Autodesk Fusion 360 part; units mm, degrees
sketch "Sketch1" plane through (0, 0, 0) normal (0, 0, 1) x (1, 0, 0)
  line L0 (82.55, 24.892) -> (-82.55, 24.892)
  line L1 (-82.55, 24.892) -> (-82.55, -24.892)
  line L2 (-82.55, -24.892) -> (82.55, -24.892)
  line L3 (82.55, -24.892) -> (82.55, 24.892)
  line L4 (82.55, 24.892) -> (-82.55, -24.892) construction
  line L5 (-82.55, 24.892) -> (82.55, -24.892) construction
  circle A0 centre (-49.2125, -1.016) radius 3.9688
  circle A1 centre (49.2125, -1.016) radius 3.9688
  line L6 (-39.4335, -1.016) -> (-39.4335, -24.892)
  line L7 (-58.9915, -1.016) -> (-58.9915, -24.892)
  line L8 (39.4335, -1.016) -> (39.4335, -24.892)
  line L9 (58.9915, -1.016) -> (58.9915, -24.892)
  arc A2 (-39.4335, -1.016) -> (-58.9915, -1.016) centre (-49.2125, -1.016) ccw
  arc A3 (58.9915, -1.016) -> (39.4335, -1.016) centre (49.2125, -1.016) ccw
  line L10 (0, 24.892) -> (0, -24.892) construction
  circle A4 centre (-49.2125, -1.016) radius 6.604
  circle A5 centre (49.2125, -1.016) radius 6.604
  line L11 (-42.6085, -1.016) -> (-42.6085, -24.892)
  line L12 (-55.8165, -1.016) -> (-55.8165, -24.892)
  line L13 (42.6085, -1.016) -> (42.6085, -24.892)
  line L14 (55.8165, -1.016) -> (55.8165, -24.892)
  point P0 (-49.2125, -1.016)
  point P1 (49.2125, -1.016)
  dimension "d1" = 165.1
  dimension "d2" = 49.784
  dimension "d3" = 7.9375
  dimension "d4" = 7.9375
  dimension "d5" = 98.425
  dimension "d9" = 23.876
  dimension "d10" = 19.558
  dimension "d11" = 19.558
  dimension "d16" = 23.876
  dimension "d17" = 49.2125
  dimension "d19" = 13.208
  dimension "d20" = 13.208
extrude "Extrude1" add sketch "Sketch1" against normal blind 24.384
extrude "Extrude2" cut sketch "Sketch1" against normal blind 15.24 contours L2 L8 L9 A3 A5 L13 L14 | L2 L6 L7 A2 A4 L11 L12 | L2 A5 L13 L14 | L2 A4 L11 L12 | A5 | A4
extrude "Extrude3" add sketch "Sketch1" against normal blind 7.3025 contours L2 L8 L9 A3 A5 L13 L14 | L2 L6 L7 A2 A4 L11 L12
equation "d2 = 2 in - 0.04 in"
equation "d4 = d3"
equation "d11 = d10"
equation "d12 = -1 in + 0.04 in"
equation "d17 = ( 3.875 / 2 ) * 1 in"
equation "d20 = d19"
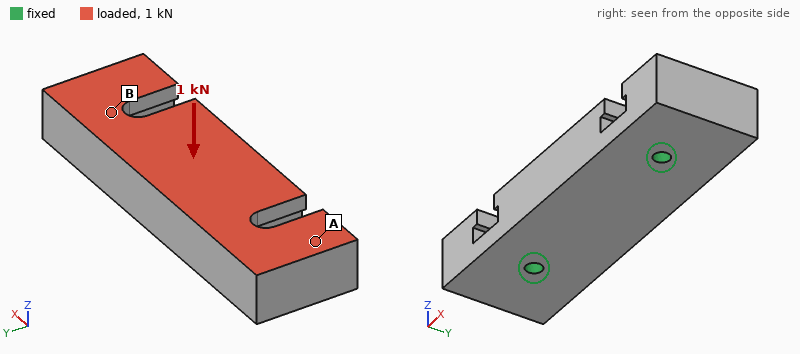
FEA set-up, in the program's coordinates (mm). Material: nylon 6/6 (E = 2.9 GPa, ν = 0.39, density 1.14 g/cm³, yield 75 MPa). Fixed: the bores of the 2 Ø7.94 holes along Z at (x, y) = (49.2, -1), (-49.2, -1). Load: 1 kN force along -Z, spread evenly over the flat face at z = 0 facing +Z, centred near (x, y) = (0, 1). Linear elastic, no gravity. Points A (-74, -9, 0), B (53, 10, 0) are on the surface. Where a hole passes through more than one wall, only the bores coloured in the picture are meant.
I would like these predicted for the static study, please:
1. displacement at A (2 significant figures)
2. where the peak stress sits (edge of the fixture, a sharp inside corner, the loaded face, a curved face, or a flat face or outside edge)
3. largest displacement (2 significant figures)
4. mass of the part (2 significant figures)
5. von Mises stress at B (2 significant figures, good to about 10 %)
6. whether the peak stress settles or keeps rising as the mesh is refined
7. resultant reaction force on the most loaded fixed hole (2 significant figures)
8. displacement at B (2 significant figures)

26 µm
edge of the fixture
46 µm
210 g
1.2 MPa
keeps rising
510 N
25 µm
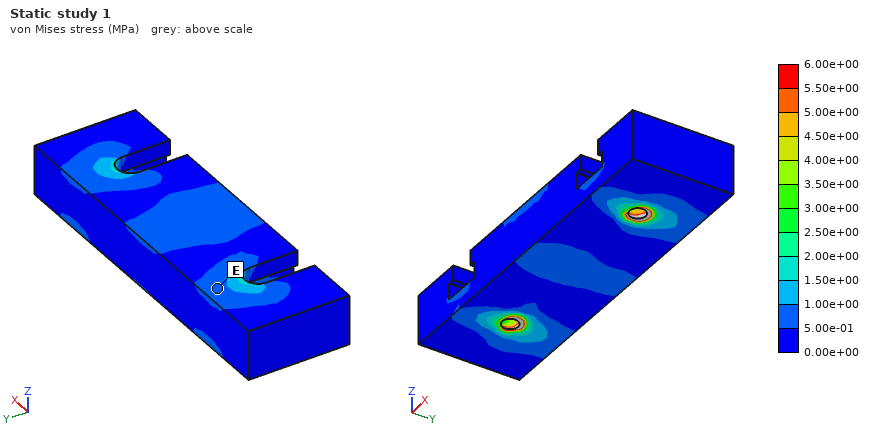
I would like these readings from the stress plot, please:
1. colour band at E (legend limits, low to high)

5.00e-01 to 1.00e+00 MPa
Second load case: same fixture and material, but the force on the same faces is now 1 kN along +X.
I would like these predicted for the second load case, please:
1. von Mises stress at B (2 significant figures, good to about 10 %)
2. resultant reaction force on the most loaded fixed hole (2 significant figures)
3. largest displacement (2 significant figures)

1.7 MPa
530 N
68 µm
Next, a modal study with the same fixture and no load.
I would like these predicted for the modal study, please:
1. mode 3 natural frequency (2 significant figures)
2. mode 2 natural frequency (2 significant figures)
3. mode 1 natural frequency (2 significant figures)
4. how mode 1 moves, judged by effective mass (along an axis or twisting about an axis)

1800 Hz
1600 Hz
1100 Hz
along Y
